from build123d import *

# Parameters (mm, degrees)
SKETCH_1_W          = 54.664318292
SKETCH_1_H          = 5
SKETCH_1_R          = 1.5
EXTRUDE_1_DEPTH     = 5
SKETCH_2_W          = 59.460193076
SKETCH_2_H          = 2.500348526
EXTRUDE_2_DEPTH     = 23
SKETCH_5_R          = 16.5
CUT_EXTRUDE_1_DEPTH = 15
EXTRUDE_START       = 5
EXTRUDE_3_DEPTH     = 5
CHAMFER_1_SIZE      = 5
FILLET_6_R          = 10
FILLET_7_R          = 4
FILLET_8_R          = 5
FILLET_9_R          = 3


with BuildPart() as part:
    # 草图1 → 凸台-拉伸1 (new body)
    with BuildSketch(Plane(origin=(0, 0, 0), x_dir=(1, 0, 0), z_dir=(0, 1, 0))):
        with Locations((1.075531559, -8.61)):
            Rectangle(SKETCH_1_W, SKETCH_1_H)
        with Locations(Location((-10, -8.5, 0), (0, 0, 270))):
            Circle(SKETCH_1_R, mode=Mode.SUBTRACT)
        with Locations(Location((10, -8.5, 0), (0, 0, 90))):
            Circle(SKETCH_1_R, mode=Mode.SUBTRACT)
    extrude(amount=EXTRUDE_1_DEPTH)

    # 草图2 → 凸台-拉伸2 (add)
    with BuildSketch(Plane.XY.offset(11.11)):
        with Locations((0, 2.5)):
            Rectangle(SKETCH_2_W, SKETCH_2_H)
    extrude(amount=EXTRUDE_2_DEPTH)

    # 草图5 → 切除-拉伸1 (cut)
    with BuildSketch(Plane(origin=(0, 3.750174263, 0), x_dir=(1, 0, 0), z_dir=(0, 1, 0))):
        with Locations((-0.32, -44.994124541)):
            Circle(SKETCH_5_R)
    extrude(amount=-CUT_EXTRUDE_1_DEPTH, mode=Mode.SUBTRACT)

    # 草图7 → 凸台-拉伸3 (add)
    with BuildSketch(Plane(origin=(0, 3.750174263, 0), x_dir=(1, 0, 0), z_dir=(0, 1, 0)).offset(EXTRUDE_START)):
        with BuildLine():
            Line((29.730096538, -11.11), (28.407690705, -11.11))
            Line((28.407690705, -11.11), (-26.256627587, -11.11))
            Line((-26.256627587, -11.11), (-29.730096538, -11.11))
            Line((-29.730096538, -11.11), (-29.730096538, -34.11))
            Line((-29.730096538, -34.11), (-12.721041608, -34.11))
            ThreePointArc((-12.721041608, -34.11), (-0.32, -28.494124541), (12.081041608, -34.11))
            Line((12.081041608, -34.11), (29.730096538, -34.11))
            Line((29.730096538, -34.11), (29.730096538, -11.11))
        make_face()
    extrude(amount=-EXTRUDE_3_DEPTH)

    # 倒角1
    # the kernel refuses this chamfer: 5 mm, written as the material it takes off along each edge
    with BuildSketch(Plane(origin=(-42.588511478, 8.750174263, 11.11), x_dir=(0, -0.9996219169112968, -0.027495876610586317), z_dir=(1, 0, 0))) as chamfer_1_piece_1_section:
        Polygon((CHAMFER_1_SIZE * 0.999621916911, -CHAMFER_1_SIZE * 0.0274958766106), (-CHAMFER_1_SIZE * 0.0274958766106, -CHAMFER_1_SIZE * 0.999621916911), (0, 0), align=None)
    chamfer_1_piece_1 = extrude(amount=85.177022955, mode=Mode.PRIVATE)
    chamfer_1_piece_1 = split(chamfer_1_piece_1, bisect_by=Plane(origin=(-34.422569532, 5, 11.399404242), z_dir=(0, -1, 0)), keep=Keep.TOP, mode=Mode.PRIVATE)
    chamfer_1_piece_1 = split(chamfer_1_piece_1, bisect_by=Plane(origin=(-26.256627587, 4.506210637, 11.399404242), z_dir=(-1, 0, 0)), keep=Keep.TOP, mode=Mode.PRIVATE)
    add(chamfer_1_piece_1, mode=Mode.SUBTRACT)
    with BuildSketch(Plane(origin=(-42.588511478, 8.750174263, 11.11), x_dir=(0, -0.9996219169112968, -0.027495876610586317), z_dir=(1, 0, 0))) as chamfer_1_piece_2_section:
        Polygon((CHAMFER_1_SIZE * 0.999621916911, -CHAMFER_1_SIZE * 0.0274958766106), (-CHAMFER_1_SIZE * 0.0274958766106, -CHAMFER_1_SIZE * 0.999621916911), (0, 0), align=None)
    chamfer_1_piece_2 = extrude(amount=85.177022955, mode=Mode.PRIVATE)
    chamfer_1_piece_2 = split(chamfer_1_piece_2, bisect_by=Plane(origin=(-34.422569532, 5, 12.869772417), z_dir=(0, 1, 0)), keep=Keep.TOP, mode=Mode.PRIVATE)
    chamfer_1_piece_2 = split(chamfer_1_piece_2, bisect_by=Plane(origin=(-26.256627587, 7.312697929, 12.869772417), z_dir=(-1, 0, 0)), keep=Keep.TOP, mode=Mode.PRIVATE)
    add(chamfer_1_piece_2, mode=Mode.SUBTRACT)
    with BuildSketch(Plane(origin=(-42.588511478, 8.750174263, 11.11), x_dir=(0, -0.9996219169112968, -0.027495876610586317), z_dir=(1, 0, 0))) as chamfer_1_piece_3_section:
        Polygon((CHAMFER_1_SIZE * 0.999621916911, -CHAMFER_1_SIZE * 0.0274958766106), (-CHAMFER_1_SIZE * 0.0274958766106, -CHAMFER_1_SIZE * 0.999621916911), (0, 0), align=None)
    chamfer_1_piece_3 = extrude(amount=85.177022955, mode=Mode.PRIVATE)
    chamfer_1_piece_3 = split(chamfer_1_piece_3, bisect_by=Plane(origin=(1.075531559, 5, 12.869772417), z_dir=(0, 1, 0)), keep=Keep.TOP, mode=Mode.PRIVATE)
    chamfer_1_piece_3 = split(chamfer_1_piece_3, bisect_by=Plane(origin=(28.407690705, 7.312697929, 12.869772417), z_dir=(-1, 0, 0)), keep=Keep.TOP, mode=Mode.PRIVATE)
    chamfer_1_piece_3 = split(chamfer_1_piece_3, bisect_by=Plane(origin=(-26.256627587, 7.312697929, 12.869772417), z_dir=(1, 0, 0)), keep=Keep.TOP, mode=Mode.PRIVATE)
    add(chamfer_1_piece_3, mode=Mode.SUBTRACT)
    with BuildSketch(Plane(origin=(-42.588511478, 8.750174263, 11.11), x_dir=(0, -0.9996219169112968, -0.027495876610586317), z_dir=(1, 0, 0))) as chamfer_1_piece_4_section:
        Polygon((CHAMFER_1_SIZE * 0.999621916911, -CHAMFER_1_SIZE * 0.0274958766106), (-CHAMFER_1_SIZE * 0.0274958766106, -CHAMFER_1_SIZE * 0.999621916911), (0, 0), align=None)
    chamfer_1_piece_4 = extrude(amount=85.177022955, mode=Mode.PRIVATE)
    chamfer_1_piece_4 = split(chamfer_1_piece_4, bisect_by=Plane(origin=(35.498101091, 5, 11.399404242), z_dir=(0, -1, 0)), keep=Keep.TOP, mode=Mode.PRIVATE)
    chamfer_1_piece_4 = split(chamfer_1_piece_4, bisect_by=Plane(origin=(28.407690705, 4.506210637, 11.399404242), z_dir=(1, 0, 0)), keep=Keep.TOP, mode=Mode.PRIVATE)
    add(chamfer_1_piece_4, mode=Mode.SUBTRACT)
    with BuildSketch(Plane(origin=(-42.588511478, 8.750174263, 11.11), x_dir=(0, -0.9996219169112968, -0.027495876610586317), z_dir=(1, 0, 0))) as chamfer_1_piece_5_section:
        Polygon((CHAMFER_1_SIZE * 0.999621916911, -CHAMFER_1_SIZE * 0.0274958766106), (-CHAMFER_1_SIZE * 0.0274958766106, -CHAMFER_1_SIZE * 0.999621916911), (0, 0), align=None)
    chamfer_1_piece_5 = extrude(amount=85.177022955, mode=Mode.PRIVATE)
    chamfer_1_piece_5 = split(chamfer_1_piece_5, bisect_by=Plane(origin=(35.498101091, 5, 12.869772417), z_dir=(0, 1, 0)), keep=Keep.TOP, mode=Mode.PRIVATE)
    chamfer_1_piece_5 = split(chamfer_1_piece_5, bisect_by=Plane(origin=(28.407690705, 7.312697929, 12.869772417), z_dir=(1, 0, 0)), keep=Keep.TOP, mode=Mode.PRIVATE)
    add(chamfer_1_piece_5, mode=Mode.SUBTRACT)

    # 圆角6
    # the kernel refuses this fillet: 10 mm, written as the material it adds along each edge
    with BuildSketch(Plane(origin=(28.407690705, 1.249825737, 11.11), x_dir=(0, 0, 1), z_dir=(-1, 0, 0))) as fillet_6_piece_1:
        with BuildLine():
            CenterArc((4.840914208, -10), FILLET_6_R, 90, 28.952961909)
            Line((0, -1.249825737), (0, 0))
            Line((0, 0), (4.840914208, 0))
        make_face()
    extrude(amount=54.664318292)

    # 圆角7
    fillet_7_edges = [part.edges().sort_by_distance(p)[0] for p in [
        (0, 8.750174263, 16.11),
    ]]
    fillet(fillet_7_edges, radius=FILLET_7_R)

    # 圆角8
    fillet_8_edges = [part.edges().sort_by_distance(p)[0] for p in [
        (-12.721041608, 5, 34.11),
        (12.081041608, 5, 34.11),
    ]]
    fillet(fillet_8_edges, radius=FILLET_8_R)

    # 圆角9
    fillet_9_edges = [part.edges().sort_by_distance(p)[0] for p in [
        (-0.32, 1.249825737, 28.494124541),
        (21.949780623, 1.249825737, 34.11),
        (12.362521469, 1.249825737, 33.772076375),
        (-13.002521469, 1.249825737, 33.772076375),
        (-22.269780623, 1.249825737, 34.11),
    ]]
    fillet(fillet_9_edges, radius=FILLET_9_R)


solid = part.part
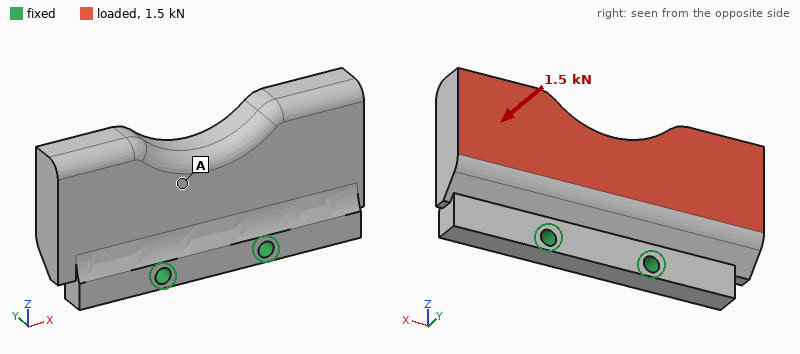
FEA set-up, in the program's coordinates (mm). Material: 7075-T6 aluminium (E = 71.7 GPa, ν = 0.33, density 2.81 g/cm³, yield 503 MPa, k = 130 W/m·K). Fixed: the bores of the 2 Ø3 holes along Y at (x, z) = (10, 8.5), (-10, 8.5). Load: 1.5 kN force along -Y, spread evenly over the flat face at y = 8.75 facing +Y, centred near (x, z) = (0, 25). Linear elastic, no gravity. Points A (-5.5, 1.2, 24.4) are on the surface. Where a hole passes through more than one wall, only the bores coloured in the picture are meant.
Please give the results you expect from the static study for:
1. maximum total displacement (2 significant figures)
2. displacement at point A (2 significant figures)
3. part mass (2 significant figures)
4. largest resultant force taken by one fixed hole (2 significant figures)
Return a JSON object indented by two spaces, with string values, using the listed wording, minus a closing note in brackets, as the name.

{
  "maximum total displacement": "0.21 mm",
  "displacement at point A": "0.10 mm",
  "part mass": "28 g",
  "largest resultant force taken by one fixed hole": "760 N"
}
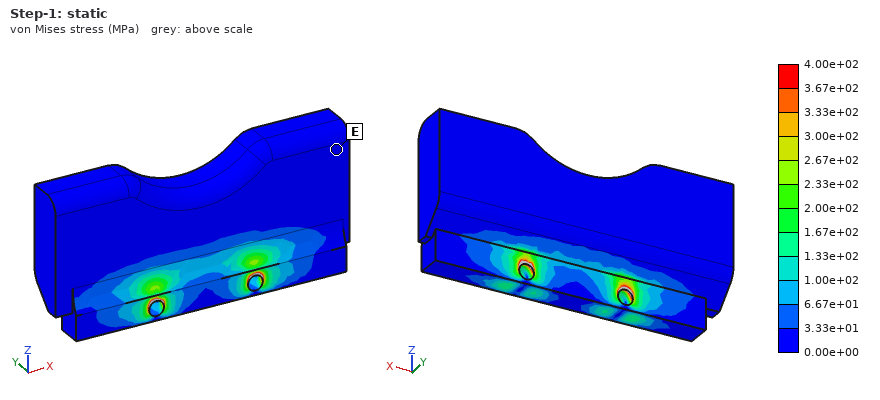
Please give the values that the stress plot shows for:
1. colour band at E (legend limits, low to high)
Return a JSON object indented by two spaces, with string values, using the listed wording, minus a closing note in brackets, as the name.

{
  "colour band at E": "0.00e+00 to 3.33e+01 MPa"
}
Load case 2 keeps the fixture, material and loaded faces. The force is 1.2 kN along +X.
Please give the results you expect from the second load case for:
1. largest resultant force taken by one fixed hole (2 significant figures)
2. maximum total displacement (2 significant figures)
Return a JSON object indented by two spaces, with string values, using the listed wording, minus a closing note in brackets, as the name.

{
  "largest resultant force taken by one fixed hole": "1.1 kN",
  "maximum total displacement": "25 µm"
}
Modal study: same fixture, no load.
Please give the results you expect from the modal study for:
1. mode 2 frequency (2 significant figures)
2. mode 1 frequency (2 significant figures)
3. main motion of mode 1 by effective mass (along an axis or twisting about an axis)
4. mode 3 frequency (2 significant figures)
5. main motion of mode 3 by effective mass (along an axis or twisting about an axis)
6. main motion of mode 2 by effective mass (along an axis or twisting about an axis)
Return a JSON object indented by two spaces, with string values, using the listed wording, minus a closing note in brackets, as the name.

{
  "mode 2 frequency": "5100 Hz",
  "mode 1 frequency": "3900 Hz",
  "main motion of mode 1 by effective mass": "along Y",
  "mode 3 frequency": "10 kHz",
  "main motion of mode 3 by effective mass": "along X",
  "main motion of mode 2 by effective mass": "twisting about Z"
}
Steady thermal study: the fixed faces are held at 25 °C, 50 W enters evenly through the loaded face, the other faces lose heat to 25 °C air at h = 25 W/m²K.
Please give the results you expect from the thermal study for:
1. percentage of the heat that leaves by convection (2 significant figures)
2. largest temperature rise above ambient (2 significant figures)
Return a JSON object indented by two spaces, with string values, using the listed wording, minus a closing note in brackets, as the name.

{
  "percentage of the heat that leaves by convection": "3.4 %",
  "largest temperature rise above ambient": "32 K"
}
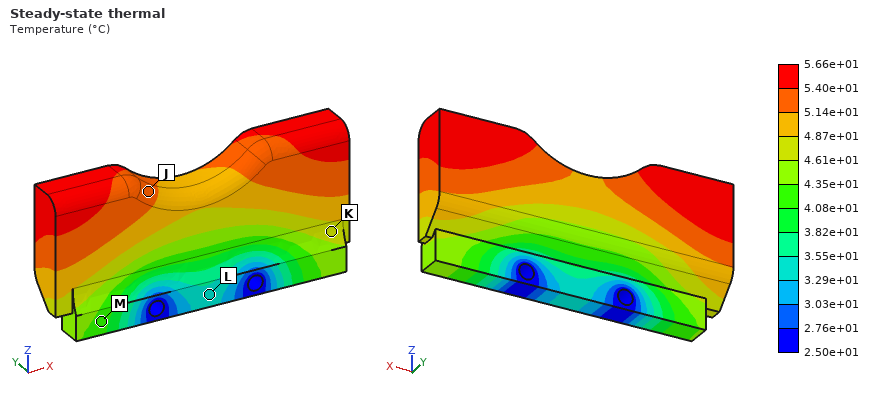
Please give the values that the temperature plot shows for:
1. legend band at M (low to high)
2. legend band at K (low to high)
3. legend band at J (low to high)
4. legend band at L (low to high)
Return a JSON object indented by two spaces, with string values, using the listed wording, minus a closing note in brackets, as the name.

{
  "legend band at M": "4.08e+01 to 4.35e+01 °C",
  "legend band at K": "4.61e+01 to 4.87e+01 °C",
  "legend band at J": "5.14e+01 to 5.40e+01 °C",
  "legend band at L": "3.29e+01 to 3.55e+01 °C"
}
